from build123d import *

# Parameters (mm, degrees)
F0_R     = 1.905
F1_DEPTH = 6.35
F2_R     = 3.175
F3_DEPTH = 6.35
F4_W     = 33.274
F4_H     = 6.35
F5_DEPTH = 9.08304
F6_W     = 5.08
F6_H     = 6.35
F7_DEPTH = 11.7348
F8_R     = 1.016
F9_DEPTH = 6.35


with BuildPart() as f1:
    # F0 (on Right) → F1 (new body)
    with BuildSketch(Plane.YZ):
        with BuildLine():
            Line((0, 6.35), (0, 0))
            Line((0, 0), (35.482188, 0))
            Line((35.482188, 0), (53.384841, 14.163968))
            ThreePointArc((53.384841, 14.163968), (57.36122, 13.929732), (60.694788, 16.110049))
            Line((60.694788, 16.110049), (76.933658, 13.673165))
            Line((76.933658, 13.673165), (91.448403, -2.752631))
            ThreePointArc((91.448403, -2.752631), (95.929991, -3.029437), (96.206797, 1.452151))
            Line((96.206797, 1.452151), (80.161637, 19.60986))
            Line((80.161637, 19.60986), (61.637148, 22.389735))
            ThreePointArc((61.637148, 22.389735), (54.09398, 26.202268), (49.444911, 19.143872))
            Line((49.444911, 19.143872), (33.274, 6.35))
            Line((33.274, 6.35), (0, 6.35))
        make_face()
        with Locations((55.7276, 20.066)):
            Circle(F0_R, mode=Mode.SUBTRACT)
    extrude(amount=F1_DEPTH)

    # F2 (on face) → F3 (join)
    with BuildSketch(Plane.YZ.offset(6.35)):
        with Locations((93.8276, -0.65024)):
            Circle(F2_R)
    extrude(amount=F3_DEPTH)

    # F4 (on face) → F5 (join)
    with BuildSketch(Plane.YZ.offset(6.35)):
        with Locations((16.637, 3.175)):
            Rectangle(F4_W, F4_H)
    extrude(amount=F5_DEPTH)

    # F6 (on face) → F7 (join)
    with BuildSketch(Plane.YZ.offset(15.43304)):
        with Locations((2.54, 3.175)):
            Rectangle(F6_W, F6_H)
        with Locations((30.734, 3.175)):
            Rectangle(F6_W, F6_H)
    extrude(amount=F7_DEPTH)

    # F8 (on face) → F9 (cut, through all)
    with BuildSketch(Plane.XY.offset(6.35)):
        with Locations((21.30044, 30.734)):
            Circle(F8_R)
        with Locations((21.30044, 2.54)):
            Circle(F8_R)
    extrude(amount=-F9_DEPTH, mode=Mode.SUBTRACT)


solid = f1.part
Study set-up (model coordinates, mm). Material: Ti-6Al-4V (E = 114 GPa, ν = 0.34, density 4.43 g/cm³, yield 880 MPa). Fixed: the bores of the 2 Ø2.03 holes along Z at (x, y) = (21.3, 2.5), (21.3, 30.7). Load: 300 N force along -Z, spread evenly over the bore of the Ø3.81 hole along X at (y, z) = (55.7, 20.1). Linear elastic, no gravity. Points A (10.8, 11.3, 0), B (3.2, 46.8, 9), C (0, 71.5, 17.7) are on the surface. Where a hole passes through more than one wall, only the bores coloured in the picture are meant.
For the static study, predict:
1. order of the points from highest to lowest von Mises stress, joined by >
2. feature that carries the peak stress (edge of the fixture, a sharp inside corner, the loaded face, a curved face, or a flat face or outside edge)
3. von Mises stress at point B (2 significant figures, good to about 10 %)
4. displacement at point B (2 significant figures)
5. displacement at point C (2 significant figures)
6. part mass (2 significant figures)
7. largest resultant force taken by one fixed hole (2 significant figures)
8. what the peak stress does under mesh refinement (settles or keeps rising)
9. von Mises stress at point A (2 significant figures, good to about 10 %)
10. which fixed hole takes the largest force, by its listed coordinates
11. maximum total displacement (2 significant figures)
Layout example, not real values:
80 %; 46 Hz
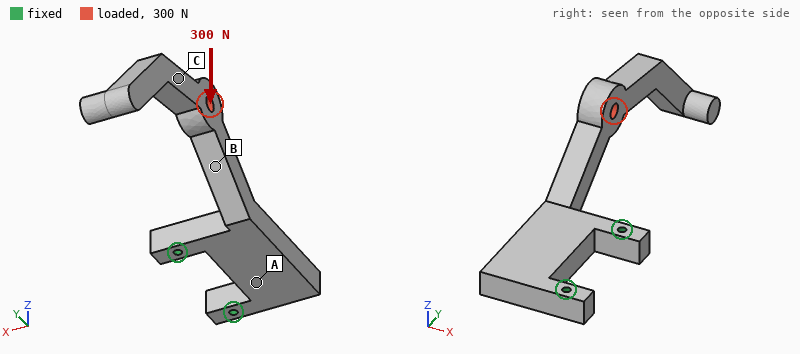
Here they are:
B > A > C; edge of the fixture; 81 MPa; 0.16 mm; 0.44 mm; 33 g; 530 N; keeps rising; 37 MPa; (21.3, 30.7); 0.70 mm
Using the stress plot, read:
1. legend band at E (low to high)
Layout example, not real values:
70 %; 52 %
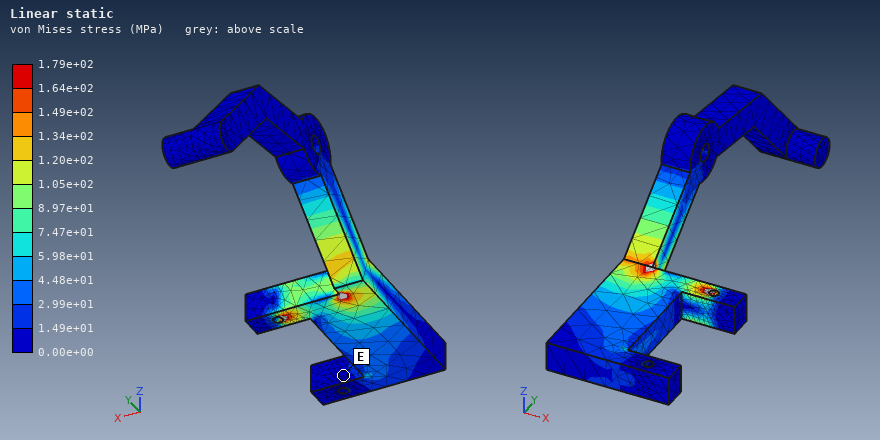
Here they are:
0.00e+00 to 1.49e+01 MPa
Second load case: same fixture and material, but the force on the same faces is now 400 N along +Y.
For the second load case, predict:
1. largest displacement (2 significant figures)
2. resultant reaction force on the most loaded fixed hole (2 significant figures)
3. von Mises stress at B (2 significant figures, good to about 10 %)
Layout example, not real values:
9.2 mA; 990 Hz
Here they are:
0.62 mm; 360 N; 73 MPa
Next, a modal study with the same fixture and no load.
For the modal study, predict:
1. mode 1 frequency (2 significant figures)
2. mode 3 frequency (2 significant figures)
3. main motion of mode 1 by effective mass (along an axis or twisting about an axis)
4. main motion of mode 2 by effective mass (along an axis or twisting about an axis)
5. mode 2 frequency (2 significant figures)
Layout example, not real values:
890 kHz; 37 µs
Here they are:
740 Hz; 2200 Hz; along Z; along X; 790 Hz
